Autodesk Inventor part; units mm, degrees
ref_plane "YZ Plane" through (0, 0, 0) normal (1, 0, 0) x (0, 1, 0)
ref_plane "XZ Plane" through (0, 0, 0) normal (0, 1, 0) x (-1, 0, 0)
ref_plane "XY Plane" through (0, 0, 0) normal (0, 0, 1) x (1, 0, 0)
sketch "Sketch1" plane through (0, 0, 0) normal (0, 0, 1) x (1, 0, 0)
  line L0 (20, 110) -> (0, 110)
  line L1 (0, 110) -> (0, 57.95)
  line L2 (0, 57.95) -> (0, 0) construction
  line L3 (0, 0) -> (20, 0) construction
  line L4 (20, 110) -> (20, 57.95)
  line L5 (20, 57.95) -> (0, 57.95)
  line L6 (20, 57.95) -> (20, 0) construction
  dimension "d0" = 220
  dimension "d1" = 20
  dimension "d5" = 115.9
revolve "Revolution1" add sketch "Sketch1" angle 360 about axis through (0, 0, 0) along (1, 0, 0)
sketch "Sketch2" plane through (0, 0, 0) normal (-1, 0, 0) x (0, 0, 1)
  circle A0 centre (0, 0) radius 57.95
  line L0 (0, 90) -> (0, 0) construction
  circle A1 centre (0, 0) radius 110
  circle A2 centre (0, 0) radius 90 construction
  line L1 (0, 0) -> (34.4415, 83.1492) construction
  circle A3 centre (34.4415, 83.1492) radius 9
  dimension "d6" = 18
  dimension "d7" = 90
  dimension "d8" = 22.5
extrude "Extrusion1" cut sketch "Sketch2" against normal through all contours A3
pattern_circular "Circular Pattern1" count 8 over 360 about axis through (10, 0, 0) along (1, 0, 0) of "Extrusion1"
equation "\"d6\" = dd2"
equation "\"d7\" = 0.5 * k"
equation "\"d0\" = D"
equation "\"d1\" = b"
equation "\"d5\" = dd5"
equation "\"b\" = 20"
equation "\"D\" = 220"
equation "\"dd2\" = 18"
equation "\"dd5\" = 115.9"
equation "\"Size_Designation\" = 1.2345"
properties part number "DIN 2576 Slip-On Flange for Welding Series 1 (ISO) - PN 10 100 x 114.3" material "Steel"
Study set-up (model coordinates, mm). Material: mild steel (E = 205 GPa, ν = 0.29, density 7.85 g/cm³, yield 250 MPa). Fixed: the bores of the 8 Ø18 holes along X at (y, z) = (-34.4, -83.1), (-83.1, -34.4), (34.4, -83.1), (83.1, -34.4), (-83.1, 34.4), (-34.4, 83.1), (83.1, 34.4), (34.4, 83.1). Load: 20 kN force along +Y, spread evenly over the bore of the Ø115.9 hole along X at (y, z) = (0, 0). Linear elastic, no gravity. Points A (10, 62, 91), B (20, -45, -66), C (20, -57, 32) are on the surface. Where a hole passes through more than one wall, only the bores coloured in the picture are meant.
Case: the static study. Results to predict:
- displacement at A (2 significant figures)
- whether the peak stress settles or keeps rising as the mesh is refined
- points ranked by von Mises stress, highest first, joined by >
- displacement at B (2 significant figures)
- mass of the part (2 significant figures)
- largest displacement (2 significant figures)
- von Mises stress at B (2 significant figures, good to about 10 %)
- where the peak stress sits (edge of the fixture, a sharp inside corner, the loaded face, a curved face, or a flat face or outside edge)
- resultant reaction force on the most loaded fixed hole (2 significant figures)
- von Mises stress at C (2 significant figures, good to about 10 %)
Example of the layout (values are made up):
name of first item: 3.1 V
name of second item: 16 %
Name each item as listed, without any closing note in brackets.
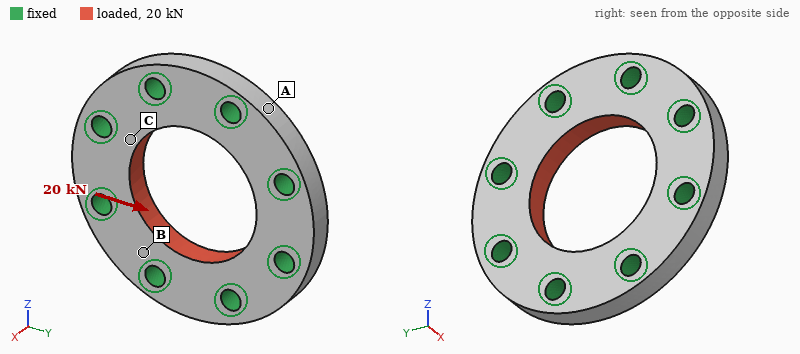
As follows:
displacement at A: 0.12 µm
whether the peak stress settles or keeps rising as the mesh is refined: keeps rising
points ranked by von Mises stress, highest first, joined by >: C > B > A
displacement at B: 0.25 µm
mass of the part: 4.0 kg
largest displacement: 0.67 µm
von Mises stress at B: 1.5 MPa
where the peak stress sits: edge of the fixture
resultant reaction force on the most loaded fixed hole: 3.2 kN
von Mises stress at C: 3.9 MPa
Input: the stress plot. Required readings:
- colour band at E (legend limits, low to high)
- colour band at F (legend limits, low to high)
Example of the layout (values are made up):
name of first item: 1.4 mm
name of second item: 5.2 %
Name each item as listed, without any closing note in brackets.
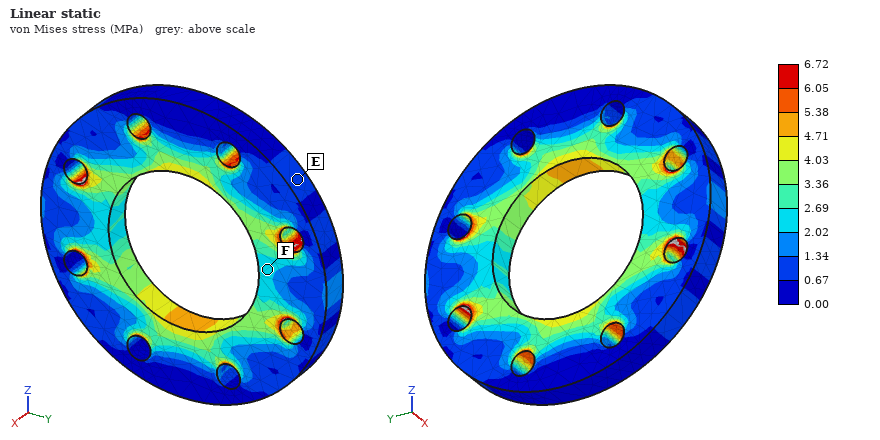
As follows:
colour band at E: 0.67 to 1.34 MPa
colour band at F: 2.02 to 2.69 MPa
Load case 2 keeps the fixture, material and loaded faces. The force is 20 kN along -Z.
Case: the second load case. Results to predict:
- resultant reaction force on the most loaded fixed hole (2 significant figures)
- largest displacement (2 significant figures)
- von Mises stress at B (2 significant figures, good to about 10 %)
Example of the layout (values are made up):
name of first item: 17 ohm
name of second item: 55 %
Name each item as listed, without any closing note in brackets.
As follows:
resultant reaction force on the most loaded fixed hole: 3.2 kN
largest displacement: 0.67 µm
von Mises stress at B: 2.6 MPa
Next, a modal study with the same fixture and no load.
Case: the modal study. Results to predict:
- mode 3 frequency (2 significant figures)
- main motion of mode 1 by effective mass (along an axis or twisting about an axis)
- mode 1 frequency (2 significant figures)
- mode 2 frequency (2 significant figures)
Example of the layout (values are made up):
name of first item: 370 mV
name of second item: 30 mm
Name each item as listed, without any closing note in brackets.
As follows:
mode 3 frequency: 15 kHz
main motion of mode 1 by effective mass: along X
mode 1 frequency: 15 kHz
mode 2 frequency: 15 kHz
